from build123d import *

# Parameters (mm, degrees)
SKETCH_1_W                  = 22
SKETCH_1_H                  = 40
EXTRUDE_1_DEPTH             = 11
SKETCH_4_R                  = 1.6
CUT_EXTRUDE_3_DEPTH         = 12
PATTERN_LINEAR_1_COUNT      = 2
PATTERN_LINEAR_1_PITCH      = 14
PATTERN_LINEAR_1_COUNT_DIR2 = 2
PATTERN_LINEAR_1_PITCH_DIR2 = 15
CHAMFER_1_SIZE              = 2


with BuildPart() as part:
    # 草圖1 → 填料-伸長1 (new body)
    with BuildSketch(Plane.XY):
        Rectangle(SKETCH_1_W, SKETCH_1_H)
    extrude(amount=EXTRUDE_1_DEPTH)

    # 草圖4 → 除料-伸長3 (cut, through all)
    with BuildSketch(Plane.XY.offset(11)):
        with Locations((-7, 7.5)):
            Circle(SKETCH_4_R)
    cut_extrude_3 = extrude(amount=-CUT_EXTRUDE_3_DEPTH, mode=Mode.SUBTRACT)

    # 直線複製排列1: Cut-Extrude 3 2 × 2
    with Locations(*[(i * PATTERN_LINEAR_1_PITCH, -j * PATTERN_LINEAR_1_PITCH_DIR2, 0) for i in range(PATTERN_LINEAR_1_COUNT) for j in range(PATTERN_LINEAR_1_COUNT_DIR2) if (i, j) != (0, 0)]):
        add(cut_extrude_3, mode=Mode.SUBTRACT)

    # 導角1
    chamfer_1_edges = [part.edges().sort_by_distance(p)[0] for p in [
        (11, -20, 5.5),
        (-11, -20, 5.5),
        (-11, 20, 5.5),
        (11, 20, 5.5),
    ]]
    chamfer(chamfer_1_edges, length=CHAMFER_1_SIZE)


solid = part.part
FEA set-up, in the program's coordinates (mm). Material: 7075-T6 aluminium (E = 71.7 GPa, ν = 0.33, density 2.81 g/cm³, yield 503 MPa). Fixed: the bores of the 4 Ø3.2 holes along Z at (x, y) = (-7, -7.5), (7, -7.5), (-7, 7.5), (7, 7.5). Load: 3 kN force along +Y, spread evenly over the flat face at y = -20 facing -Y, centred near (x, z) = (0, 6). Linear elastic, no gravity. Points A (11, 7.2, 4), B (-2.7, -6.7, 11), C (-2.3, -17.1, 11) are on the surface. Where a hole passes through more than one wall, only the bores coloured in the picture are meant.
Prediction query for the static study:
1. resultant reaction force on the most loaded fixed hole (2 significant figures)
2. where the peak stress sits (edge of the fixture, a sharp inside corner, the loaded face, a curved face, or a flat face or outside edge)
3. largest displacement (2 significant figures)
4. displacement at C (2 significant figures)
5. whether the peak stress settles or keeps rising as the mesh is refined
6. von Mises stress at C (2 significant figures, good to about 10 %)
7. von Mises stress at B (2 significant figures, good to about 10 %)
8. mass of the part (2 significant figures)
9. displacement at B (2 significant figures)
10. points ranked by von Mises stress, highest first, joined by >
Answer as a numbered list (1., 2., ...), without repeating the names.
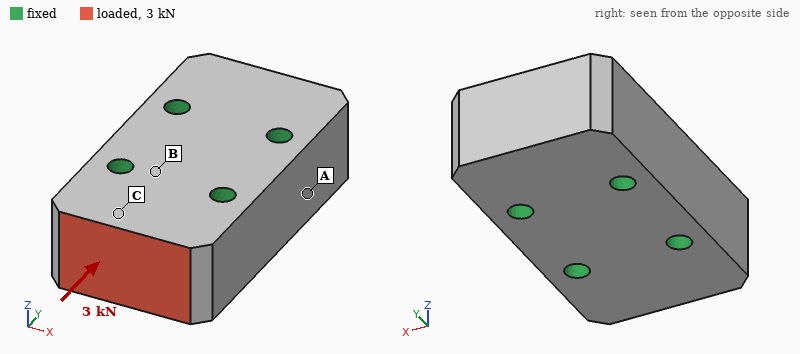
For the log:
1. 1.4 kN
2. edge of the fixture
3. 2.8 µm
4. 2.2 µm
5. keeps rising
6. 14 MPa
7. 6.9 MPa
8. 26 g
9. 0.62 µm
10. C > B > A
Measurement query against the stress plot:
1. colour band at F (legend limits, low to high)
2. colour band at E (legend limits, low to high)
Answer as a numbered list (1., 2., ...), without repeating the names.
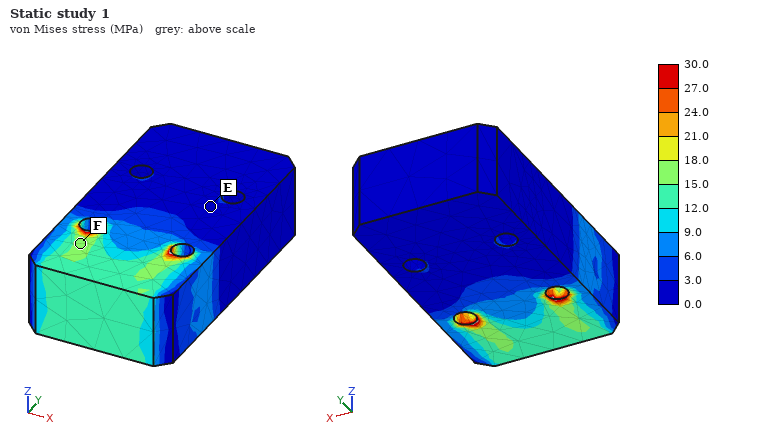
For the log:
1. 15.0 to 18.0 MPa
2. 0.0 to 3.0 MPa
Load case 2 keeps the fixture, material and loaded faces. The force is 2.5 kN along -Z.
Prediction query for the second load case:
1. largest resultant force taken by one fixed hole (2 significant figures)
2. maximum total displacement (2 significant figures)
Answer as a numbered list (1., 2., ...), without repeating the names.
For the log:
1. 1.4 kN
2. 19 µm
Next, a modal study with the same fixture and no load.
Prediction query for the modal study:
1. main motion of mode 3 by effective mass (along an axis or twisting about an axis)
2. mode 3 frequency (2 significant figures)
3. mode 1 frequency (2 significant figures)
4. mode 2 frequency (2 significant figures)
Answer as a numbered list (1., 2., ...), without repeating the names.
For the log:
1. twisting about Z
2. 52 kHz
3. 39 kHz
4. 40 kHz
